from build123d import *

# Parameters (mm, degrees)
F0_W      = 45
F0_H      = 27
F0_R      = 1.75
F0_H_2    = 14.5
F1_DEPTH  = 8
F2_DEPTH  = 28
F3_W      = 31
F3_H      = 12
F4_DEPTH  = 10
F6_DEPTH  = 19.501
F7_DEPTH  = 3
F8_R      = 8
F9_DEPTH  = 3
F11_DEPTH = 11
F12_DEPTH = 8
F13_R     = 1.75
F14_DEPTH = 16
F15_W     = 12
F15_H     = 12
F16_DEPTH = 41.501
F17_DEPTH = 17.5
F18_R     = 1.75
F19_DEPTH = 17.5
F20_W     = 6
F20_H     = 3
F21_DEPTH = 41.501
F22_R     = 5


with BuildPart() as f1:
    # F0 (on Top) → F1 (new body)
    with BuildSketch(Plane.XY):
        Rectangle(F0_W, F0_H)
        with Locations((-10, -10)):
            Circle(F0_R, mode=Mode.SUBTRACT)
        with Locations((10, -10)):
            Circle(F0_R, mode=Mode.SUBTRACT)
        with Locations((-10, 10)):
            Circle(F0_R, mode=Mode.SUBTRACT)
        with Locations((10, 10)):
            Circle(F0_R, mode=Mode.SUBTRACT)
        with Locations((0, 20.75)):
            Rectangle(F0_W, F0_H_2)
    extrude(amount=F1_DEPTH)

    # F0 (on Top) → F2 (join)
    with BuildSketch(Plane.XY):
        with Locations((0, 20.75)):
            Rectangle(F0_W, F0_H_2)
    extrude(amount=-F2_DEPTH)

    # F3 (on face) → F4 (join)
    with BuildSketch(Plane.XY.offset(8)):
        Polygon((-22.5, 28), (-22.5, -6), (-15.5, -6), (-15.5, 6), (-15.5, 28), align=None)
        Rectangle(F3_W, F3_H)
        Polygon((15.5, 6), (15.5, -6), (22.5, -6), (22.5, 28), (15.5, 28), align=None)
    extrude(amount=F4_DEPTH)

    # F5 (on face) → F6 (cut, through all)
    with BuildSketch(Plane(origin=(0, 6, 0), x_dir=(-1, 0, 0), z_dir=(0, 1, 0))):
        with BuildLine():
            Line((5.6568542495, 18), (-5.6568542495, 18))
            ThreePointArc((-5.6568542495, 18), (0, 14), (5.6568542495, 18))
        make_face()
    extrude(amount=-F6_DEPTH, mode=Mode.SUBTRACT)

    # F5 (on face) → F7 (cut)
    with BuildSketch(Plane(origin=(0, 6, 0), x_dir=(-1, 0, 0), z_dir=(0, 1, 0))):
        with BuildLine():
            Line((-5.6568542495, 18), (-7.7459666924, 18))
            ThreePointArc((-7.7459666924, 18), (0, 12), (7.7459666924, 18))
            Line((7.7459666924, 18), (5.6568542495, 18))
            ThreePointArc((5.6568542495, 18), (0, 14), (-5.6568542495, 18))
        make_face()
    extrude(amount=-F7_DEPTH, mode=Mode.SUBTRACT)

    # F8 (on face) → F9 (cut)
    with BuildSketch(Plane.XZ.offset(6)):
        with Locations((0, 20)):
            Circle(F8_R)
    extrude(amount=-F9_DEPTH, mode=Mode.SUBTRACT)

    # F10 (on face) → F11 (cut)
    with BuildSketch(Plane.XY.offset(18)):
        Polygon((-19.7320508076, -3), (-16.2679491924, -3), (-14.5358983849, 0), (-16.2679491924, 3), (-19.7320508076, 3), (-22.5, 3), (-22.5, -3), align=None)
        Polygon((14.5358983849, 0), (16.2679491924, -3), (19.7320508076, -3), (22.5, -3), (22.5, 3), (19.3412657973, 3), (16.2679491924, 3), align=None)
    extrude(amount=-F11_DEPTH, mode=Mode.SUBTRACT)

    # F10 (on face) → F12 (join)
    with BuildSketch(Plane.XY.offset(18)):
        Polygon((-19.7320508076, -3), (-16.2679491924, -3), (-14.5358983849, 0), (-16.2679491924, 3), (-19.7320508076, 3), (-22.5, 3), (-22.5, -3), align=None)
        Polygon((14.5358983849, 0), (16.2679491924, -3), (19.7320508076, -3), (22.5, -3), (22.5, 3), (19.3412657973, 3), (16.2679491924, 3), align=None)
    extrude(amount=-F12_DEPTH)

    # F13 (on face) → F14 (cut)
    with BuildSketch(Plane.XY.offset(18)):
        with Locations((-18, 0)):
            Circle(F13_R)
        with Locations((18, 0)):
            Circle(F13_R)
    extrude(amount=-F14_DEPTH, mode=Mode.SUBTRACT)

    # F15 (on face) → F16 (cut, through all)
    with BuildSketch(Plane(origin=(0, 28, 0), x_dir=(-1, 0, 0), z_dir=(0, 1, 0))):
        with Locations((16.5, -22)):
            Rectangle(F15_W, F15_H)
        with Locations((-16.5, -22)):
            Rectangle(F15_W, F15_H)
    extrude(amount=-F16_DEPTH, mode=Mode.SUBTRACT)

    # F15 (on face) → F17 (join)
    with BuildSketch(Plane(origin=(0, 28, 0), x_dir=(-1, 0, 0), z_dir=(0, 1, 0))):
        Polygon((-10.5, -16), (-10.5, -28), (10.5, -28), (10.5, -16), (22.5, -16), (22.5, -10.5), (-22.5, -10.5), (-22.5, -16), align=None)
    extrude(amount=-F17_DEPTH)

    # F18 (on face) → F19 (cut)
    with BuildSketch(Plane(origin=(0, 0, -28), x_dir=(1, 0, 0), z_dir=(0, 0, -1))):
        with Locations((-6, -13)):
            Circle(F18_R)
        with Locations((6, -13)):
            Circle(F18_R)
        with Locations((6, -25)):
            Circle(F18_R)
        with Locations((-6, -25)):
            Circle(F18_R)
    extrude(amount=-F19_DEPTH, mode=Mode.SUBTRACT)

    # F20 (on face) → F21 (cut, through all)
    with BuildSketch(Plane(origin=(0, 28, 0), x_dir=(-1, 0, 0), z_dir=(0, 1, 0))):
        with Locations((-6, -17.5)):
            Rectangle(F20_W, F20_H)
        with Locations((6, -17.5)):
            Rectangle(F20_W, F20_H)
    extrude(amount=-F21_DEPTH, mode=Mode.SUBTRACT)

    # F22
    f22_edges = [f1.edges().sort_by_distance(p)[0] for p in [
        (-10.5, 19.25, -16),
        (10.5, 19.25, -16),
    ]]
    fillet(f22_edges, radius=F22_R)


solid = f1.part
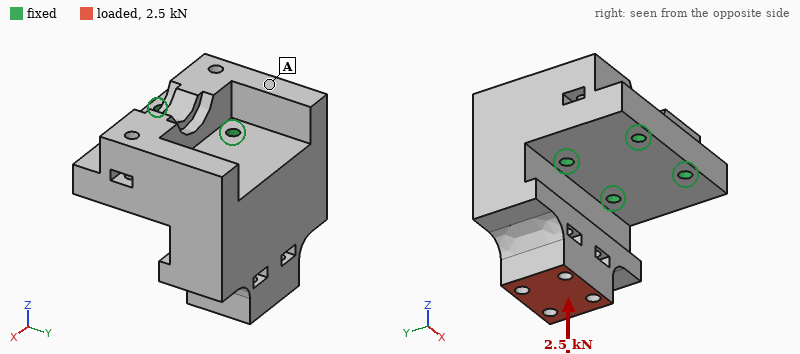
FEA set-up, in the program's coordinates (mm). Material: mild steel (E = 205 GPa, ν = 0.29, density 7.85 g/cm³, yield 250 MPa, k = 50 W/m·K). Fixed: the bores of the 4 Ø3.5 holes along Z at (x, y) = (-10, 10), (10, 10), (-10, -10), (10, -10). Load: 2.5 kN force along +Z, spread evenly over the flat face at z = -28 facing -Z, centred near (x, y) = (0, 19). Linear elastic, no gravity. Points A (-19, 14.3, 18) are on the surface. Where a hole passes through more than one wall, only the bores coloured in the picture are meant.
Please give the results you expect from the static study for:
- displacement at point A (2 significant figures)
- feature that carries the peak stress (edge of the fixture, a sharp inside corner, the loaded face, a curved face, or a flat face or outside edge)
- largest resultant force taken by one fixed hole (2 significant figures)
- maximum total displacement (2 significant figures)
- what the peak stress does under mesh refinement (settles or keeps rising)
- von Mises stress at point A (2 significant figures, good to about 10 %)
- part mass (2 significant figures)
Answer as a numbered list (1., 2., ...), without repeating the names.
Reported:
1. 2.4 µm
2. edge of the fixture
3. 1.6 kN
4. 8.4 µm
5. keeps rising
6. 8.7 MPa
7. 290 g
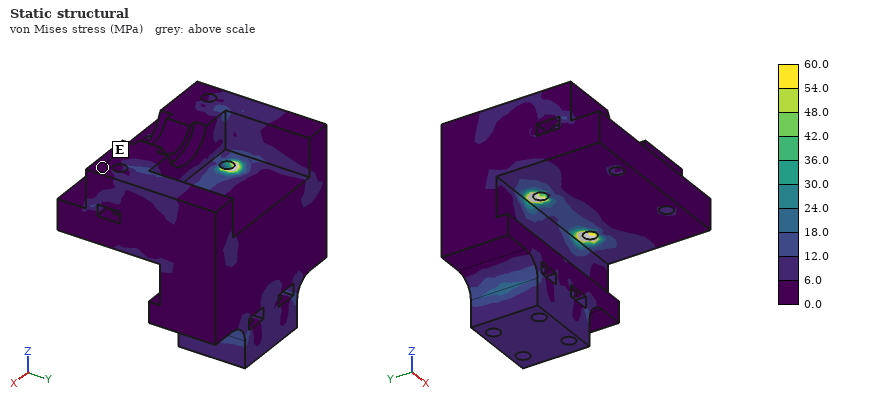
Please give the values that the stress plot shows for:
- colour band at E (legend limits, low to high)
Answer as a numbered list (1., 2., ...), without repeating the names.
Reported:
1. 0.0 to 6.0 MPa
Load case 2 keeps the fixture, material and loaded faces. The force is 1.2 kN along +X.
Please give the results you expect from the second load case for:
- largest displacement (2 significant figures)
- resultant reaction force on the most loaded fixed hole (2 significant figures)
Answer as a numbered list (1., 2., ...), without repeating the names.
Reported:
1. 7.7 µm
2. 1.7 kN
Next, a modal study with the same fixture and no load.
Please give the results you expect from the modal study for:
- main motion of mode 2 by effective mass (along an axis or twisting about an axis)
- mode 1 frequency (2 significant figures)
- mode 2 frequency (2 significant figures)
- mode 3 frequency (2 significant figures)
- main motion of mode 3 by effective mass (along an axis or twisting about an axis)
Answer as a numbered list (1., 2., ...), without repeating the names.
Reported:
1. along X
2. 5900 Hz
3. 9300 Hz
4. 15 kHz
5. along X
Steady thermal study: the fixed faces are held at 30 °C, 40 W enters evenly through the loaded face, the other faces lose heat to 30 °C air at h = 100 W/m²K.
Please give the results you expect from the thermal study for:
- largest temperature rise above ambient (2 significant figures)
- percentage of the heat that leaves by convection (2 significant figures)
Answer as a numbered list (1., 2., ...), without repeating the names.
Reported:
1. 66 K
2. 42 %
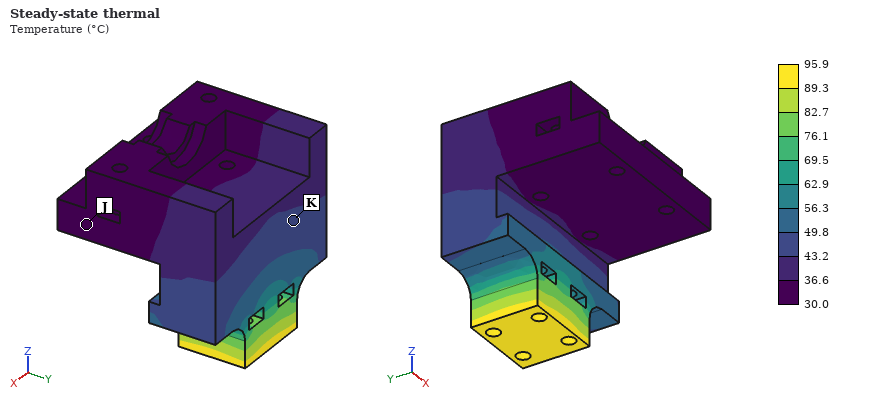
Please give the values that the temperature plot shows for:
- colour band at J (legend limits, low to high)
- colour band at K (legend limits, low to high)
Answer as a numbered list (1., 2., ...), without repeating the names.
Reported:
1. 30.0 to 36.6 °C
2. 43.2 to 49.8 °C
